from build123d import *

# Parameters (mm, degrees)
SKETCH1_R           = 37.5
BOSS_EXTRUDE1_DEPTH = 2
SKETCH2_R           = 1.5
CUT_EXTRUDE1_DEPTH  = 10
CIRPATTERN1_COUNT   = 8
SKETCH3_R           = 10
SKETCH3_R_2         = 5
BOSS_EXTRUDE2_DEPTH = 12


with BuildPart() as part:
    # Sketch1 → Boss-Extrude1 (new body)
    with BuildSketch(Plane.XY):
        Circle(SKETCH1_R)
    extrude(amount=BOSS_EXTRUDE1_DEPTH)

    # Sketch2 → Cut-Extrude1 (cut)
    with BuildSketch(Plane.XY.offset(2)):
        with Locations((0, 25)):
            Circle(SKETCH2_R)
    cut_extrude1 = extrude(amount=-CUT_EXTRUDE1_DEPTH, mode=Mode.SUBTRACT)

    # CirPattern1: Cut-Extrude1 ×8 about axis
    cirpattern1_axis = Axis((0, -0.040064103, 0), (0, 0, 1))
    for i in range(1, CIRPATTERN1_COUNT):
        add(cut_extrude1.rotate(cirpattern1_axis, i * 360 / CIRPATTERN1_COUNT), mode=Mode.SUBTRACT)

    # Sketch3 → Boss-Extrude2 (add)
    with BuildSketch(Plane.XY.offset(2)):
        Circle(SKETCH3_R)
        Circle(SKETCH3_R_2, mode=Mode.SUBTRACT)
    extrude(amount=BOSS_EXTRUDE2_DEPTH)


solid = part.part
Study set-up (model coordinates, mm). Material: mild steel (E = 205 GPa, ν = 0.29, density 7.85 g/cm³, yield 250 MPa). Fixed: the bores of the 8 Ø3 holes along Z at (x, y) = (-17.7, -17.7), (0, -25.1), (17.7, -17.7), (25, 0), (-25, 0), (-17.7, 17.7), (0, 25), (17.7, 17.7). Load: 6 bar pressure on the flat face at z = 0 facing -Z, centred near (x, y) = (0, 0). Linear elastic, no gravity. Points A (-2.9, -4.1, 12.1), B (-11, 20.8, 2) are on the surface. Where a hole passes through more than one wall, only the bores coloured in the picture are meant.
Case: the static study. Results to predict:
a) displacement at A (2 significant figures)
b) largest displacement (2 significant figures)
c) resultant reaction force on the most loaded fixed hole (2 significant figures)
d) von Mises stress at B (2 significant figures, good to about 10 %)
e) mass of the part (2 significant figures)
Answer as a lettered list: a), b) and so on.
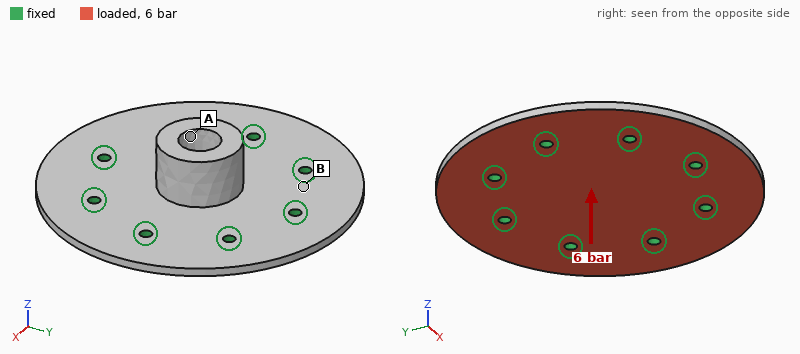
a) 10 µm
b) 16 µm
c) 330 N
d) 42 MPa
e) 91 g
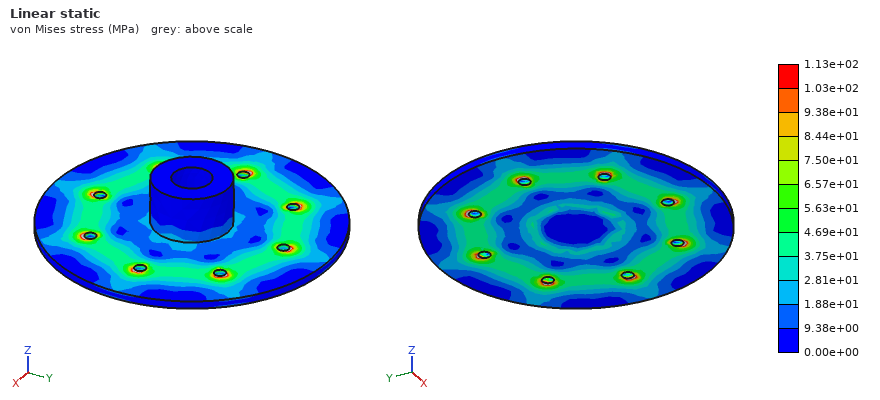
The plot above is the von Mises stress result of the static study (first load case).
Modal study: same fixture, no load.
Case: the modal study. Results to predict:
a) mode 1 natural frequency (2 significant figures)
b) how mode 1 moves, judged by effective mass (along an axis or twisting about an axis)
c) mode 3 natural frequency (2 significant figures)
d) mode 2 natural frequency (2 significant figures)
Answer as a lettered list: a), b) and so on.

a) 5600 Hz
b) along Z
c) 7900 Hz
d) 7900 Hz
